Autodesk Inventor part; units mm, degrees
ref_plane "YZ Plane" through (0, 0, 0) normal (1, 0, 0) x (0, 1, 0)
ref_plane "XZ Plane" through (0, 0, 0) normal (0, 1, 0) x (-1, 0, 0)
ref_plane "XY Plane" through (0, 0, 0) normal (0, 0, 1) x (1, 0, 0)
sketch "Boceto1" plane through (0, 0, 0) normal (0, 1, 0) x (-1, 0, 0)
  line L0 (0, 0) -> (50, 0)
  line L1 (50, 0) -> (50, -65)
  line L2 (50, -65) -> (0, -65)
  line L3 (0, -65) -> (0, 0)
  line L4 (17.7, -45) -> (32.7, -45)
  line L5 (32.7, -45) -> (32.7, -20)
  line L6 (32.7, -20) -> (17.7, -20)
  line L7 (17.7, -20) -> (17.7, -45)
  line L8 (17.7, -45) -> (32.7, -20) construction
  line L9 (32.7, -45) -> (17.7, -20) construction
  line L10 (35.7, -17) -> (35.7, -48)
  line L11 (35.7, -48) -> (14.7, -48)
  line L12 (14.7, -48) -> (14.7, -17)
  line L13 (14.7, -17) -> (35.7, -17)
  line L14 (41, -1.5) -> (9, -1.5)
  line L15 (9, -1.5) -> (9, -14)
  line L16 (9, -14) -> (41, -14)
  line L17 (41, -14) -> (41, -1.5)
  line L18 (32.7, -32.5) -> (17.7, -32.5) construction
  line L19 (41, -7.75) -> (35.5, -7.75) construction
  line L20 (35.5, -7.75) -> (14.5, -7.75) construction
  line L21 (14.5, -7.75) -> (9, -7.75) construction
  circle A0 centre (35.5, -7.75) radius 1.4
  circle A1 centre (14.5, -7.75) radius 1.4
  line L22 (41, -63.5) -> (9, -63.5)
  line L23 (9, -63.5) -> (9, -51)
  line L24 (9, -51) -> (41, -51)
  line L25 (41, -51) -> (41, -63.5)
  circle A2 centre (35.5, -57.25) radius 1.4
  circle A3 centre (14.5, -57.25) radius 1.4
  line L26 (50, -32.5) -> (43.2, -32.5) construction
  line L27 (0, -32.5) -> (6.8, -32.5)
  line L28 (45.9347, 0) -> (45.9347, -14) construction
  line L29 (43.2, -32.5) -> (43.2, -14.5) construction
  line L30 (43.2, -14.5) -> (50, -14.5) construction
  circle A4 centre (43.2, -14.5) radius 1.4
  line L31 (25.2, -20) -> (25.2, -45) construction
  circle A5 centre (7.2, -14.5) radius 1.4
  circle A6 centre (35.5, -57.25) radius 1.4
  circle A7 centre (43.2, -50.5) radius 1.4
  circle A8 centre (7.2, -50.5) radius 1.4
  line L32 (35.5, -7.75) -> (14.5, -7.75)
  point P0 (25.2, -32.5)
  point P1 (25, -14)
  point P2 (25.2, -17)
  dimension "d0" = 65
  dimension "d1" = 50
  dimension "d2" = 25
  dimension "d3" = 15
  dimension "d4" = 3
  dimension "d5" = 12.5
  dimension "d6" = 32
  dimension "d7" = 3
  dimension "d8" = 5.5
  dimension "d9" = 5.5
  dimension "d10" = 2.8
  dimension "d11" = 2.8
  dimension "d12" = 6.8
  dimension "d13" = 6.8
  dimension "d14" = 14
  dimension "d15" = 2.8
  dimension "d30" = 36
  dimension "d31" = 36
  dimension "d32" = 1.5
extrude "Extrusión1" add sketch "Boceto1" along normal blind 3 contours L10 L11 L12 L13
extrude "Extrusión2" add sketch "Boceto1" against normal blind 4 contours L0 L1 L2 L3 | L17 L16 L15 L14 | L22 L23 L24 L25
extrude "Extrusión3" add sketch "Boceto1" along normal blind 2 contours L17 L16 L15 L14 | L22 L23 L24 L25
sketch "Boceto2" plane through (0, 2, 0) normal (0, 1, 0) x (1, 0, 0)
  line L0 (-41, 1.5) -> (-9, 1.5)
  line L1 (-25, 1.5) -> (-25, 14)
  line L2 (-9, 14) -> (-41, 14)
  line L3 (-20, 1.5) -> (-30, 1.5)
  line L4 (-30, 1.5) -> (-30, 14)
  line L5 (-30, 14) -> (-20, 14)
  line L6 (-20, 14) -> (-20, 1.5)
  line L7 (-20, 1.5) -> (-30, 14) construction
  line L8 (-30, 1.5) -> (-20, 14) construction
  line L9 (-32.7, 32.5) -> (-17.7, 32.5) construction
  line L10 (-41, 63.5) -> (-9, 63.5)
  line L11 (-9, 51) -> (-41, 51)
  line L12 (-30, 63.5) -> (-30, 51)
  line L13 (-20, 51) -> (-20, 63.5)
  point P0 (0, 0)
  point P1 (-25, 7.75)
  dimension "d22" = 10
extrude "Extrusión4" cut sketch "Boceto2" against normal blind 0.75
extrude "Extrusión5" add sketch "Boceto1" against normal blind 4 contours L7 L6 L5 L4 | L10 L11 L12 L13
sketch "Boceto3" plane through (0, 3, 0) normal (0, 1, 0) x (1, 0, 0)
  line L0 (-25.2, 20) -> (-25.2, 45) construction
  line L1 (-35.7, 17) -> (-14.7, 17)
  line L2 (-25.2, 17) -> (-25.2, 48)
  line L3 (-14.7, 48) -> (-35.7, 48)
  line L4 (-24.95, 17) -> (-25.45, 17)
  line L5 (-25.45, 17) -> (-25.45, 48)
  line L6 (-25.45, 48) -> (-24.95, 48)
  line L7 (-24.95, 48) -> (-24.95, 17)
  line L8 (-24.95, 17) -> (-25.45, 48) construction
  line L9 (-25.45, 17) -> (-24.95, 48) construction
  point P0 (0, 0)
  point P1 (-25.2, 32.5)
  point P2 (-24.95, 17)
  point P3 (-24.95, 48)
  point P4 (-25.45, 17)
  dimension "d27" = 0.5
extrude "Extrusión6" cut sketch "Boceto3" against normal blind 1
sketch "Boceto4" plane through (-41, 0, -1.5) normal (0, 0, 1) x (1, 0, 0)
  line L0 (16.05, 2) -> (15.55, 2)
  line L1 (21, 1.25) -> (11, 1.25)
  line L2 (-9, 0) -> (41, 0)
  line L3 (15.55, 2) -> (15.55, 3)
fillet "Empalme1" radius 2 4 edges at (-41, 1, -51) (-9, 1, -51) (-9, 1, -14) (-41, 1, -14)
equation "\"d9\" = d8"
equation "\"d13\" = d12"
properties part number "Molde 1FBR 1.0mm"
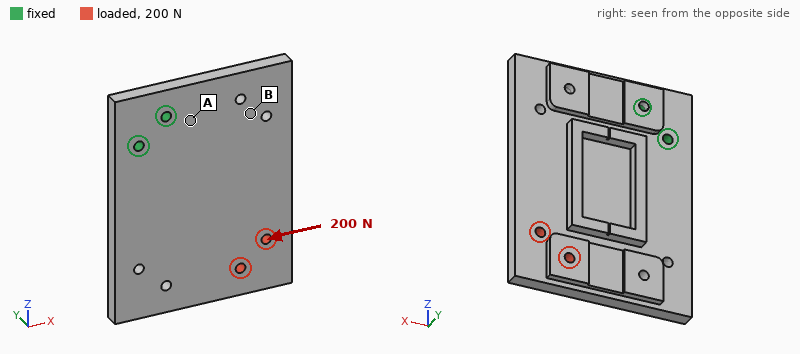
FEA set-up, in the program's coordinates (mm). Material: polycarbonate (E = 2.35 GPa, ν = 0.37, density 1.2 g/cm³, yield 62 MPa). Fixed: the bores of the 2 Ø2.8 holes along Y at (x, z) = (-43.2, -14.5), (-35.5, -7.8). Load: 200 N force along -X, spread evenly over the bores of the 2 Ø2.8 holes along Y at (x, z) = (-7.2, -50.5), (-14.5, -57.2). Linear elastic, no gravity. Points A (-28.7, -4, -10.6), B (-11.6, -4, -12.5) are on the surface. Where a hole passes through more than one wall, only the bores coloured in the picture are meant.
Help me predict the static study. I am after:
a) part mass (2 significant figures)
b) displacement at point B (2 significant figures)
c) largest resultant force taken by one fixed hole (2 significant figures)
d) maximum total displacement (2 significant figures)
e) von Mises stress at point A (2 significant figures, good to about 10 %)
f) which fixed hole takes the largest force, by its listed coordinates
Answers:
18 g
0.33 mm
770 N
0.93 mm
8.3 MPa
(-43.2, -14.5)
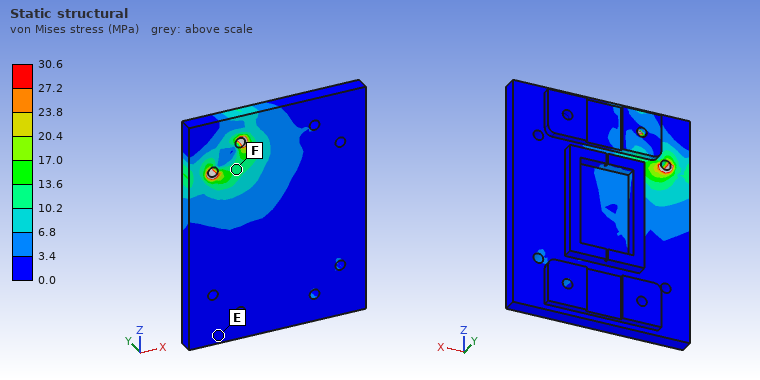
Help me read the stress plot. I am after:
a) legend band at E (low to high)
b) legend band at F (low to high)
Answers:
0.0 to 3.4 MPa
10.2 to 13.6 MPa
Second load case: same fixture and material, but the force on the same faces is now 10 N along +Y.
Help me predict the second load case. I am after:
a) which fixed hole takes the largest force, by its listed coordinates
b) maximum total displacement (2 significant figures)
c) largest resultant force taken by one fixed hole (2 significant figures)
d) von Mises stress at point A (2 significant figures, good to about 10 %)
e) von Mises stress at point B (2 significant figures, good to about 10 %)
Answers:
(-43.2, -14.5)
0.94 mm
8.9 N
3.1 MPa
1.7 MPa
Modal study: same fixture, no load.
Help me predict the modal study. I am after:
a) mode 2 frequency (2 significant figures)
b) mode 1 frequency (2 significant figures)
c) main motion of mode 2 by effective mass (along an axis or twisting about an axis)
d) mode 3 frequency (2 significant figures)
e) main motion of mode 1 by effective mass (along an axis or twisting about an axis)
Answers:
620 Hz
260 Hz
twisting about Z
910 Hz
along Y
